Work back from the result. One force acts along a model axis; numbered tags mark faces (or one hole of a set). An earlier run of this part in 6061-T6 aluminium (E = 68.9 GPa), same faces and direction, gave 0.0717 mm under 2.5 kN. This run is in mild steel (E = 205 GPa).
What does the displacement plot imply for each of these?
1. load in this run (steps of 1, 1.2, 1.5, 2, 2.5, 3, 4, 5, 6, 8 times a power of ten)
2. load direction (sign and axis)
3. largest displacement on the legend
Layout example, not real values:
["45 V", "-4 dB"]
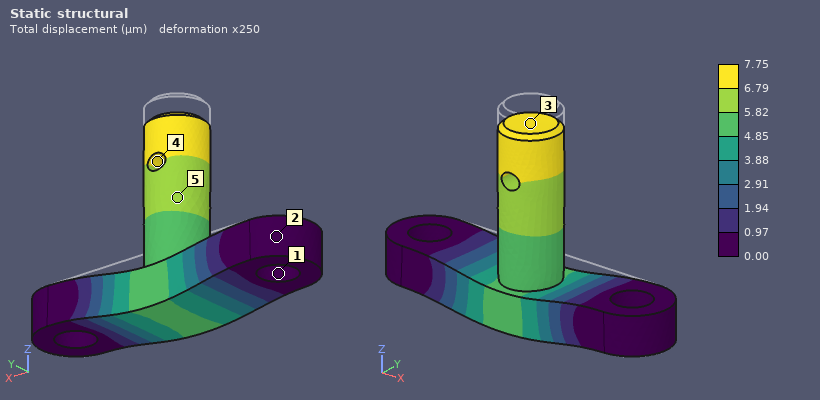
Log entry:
["800 N", "-Z", "7.75 µm"]
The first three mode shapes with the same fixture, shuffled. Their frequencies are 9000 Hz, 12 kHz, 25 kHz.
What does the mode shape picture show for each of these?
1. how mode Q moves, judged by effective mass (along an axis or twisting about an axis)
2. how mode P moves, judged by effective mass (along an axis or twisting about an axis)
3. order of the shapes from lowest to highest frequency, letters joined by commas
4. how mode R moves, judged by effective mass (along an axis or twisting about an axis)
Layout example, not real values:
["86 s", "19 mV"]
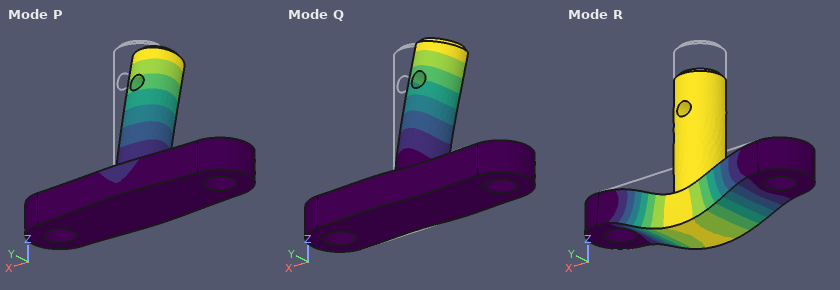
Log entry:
["along X", "along Y", "P, Q, R", "along Z"]
